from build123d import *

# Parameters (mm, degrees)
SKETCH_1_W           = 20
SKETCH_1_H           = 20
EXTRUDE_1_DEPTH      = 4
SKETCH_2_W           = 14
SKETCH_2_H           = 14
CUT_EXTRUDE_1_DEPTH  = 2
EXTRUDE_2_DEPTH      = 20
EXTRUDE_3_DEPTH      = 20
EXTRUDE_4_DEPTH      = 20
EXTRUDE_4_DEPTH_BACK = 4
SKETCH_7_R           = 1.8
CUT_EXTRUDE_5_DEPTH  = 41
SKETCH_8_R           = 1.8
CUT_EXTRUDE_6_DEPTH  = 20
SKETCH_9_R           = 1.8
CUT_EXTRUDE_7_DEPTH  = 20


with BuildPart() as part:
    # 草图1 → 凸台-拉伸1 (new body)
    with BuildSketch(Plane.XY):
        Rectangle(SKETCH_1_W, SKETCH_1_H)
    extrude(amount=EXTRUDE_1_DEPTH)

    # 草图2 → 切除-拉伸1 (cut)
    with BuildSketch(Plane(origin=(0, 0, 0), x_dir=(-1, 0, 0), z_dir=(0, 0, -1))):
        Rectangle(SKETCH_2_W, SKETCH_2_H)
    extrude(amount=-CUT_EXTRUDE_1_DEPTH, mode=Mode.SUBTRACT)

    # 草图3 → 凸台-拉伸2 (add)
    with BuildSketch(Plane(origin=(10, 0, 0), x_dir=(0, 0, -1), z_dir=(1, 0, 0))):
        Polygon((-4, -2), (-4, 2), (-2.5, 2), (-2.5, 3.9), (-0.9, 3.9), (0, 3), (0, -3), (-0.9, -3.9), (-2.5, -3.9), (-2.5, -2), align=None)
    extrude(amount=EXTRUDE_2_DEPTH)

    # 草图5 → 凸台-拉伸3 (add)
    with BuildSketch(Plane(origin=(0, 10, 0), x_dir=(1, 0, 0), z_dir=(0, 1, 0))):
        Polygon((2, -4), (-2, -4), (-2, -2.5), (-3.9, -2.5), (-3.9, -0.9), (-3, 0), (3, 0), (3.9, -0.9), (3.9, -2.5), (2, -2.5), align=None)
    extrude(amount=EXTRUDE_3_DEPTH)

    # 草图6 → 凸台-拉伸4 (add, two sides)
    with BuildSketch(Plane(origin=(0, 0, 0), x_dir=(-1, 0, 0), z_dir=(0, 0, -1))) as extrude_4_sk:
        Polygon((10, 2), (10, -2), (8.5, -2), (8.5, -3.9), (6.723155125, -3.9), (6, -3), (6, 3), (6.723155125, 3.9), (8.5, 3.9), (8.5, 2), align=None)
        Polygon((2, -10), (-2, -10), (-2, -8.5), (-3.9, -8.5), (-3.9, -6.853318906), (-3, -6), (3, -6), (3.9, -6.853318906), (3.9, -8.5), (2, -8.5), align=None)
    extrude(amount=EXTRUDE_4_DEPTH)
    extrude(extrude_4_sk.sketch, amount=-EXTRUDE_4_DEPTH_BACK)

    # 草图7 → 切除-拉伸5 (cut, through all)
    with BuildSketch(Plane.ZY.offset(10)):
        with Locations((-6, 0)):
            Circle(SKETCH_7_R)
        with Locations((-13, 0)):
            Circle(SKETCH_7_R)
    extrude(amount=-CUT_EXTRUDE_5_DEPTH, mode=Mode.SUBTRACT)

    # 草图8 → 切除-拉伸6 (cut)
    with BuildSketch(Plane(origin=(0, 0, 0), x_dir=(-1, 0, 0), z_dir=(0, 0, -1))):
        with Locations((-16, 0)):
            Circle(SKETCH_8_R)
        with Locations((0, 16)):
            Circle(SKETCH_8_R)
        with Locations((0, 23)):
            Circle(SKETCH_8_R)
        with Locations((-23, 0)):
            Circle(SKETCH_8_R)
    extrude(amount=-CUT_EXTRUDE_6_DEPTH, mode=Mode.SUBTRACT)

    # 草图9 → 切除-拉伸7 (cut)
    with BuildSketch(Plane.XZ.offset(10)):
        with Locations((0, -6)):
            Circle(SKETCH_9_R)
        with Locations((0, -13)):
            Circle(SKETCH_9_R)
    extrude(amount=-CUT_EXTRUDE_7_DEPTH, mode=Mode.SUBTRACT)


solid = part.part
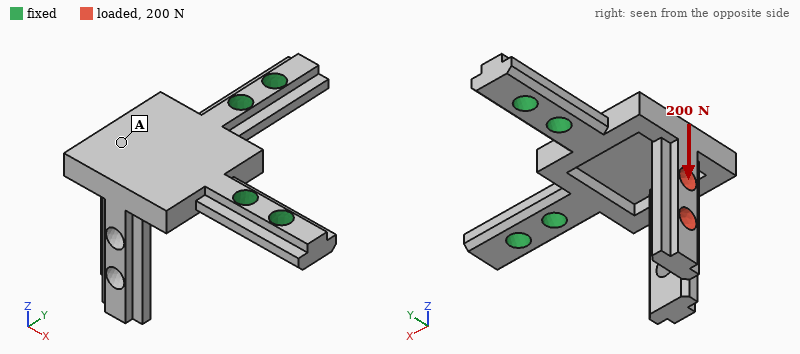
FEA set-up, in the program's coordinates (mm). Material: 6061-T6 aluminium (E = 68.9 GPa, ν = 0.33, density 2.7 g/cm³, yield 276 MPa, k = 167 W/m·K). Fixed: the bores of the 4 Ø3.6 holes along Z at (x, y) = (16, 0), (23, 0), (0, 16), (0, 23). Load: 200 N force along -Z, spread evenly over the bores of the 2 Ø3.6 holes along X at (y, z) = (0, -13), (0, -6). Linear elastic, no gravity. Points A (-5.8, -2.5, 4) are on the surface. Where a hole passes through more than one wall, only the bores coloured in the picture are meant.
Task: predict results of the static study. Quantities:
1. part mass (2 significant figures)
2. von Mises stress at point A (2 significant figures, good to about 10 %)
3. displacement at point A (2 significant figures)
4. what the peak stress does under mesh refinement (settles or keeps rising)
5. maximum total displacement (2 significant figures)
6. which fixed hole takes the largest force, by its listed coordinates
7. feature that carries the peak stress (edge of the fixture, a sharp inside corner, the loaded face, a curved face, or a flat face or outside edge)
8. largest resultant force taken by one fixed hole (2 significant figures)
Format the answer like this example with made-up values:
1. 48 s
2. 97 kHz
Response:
1. 7.8 g
2. 26 MPa
3. 0.11 mm
4. keeps rising
5. 0.27 mm
6. (0, 16)
7. edge of the fixture
8. 170 N
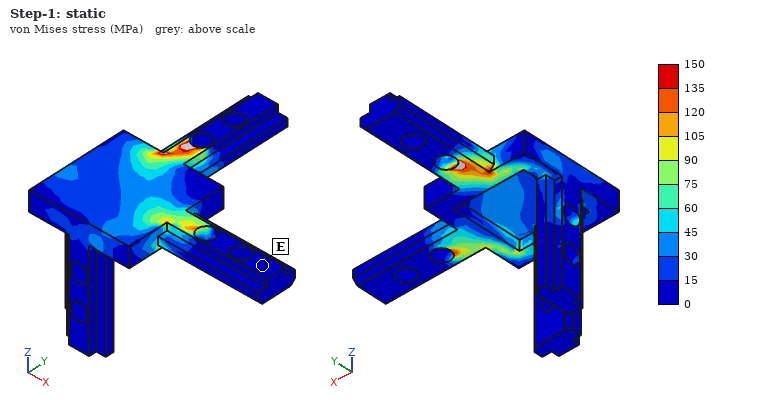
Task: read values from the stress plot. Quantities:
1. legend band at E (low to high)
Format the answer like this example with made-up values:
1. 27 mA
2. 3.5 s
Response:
1. 0 to 15 MPa
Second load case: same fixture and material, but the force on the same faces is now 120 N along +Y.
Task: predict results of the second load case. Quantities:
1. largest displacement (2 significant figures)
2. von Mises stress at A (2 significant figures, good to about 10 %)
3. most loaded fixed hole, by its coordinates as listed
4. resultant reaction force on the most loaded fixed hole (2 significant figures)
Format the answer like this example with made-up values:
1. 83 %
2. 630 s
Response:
1. 0.19 mm
2. 34 MPa
3. (0, 16)
4. 130 N
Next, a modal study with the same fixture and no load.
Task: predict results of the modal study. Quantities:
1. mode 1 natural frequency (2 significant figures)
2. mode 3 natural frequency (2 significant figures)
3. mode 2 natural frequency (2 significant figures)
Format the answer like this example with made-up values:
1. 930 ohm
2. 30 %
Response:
1. 2400 Hz
2. 4400 Hz
3. 3500 Hz
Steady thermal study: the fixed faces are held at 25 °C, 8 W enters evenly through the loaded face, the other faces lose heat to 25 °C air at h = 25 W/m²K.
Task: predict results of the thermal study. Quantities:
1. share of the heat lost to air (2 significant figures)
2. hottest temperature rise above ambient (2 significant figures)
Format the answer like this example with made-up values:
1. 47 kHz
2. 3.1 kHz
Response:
1. 10 %
2. 46 K
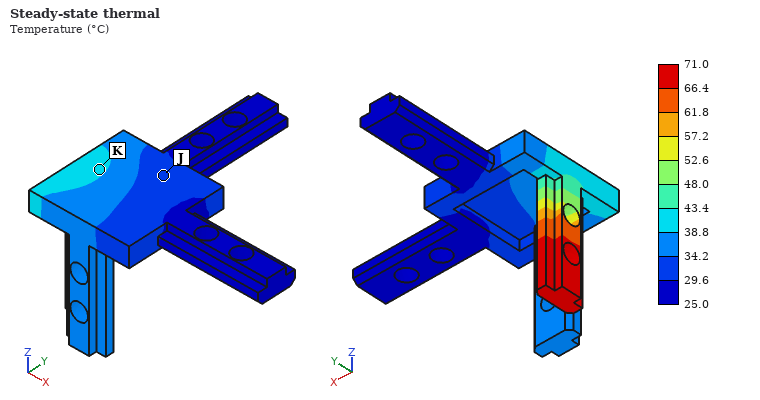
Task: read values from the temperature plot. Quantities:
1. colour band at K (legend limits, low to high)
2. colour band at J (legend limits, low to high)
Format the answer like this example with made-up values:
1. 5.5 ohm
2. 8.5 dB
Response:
1. 38.8 to 43.4 °C
2. 29.6 to 34.2 °C
